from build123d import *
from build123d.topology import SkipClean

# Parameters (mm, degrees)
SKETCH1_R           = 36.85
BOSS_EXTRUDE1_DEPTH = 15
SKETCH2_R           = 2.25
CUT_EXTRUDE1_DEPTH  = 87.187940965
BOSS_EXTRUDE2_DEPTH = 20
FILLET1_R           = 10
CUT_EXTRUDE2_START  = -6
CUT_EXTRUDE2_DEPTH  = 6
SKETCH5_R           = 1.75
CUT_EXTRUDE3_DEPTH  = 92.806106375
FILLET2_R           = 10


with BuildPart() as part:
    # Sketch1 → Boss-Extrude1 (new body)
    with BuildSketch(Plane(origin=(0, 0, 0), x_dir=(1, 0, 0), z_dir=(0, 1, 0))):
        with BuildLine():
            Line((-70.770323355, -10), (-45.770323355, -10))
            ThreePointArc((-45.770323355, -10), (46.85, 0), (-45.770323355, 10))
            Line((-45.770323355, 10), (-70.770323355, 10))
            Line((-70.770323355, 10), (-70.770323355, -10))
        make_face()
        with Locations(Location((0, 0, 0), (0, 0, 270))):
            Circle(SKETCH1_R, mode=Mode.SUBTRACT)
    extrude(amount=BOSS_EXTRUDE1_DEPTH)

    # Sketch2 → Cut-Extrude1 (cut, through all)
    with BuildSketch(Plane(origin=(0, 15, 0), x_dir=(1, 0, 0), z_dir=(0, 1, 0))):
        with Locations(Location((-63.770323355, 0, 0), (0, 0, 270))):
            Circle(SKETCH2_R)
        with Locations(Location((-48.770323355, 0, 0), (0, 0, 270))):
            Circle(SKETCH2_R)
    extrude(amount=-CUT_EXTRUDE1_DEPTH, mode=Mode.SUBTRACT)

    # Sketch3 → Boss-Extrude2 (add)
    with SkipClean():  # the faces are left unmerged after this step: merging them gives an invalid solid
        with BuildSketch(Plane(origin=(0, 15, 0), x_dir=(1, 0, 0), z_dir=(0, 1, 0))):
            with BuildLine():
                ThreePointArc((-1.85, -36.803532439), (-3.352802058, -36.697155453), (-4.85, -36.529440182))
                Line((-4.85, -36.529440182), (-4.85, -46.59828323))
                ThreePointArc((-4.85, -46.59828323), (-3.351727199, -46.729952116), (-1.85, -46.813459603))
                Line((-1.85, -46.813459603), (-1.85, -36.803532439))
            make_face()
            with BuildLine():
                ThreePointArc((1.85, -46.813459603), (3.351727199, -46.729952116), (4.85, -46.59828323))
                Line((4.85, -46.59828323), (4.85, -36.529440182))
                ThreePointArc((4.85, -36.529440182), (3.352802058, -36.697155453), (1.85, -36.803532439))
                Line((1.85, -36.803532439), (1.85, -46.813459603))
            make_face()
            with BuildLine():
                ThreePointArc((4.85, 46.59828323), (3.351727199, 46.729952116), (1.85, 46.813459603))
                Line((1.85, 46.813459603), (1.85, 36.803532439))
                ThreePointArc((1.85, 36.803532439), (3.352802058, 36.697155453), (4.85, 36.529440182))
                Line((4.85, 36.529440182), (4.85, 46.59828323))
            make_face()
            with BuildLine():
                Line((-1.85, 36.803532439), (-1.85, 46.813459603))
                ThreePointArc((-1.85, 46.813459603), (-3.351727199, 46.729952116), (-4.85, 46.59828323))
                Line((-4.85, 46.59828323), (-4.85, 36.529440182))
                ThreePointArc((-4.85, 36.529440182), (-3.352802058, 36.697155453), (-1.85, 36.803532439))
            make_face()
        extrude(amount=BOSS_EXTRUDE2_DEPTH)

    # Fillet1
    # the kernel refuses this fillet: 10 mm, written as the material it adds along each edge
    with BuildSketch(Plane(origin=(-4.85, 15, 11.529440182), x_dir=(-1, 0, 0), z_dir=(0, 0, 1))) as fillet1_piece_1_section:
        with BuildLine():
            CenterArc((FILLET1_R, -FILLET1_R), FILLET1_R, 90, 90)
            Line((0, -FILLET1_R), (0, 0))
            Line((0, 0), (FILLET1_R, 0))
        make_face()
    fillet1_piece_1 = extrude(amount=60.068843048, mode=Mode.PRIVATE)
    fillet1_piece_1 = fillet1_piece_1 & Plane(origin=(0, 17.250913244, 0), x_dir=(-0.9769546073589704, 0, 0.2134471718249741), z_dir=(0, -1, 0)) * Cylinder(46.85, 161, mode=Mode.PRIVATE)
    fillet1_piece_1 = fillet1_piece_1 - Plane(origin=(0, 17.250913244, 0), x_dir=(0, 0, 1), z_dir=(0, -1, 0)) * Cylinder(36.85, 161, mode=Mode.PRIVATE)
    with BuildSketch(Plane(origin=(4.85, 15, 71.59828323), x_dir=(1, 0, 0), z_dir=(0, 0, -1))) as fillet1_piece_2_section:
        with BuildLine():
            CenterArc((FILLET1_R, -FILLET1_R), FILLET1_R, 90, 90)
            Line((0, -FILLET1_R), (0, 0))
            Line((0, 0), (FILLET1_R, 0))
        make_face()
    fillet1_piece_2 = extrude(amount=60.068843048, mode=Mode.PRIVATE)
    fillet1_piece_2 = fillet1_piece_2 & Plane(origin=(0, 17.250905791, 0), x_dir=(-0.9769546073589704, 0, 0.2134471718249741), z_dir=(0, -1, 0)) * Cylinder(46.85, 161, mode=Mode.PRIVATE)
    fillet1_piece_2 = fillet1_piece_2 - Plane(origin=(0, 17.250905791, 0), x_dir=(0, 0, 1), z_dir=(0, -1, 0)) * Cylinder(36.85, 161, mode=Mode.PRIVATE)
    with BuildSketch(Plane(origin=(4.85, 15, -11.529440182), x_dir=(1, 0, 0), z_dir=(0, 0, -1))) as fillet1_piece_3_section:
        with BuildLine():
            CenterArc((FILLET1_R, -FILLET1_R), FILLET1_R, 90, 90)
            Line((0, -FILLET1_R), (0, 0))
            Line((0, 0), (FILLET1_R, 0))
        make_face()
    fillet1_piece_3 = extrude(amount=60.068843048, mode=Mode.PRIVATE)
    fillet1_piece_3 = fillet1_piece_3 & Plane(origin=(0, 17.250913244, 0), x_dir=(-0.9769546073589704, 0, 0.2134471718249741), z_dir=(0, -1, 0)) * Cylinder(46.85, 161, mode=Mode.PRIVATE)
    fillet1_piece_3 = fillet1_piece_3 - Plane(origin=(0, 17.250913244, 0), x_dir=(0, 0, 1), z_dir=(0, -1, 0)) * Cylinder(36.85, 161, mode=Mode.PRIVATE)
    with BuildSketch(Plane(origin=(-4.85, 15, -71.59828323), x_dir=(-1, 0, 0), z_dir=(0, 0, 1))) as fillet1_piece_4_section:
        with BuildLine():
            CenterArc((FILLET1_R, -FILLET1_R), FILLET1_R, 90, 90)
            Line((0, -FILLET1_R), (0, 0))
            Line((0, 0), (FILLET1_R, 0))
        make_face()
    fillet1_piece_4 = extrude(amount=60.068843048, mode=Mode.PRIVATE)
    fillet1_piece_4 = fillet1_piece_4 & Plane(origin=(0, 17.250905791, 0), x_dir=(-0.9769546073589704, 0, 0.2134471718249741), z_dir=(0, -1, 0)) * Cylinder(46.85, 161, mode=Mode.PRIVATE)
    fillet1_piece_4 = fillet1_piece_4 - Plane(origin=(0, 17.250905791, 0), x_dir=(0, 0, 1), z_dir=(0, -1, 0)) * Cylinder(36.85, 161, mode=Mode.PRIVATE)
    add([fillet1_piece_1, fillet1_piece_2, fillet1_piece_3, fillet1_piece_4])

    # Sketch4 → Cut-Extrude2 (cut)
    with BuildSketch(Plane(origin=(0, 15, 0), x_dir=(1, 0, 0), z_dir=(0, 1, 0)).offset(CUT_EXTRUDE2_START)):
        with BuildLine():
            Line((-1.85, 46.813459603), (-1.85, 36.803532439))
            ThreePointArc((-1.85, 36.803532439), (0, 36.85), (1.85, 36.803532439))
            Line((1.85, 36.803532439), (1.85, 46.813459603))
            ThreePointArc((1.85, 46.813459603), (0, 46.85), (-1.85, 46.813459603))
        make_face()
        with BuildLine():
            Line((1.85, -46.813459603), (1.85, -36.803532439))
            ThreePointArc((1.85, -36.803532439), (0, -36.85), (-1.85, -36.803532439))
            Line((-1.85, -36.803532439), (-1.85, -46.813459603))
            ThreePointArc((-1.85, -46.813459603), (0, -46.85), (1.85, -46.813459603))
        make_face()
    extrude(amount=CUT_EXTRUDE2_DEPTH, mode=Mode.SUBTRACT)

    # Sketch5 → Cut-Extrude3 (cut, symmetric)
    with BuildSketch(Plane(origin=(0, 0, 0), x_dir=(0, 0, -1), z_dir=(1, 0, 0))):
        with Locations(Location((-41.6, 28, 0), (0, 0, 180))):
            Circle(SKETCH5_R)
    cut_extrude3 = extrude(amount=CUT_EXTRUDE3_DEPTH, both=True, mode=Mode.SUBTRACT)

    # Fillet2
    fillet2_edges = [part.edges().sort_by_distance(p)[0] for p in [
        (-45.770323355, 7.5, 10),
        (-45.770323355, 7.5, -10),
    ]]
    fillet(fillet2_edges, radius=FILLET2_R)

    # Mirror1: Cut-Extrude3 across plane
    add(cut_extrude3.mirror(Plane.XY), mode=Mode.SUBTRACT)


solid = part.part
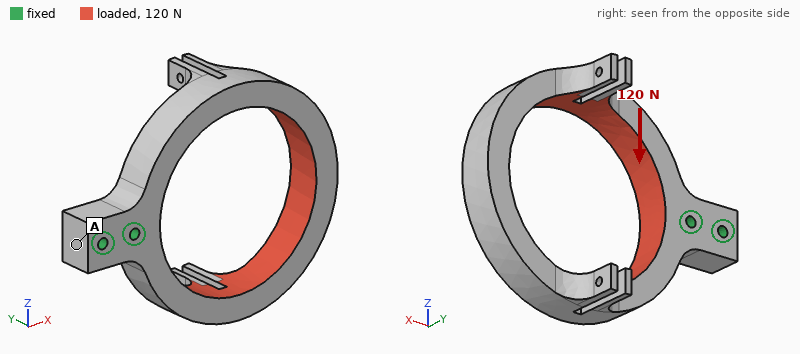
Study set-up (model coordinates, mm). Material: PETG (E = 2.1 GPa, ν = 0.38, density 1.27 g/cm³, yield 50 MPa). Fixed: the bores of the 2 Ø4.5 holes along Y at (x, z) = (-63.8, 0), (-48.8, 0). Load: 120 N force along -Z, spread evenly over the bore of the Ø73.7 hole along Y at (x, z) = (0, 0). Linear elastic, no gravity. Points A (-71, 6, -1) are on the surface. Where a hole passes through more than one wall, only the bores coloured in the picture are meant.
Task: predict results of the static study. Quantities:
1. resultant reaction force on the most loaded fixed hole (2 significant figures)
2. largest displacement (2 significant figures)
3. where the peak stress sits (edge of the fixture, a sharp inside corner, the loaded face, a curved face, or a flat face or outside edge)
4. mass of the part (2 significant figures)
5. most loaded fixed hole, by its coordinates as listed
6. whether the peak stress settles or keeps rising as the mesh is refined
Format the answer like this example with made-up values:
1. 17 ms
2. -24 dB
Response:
1. 380 N
2. 1.7 mm
3. edge of the fixture
4. 63 g
5. (-48.8, 0)
6. keeps rising
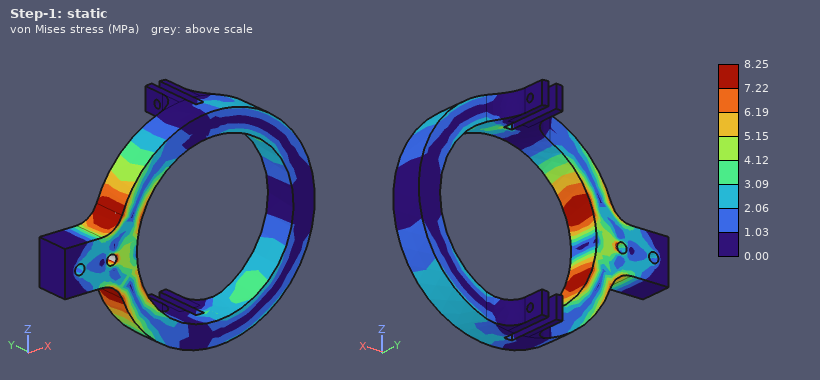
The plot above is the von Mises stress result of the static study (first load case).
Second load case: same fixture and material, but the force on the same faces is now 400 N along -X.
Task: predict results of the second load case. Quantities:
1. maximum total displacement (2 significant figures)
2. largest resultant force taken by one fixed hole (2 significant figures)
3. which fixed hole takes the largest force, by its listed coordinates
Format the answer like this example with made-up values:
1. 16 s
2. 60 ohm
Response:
1. 0.75 mm
2. 220 N
3. (-63.8, 0)
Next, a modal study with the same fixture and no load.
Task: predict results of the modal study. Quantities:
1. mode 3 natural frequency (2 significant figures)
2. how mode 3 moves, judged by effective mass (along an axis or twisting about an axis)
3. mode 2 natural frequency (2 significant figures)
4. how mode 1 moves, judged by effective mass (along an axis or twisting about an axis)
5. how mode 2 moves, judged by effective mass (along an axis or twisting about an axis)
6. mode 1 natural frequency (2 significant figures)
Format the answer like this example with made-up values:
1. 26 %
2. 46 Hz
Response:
1. 400 Hz
2. twisting about X
3. 200 Hz
4. along Y
5. along Z
6. 170 Hz
